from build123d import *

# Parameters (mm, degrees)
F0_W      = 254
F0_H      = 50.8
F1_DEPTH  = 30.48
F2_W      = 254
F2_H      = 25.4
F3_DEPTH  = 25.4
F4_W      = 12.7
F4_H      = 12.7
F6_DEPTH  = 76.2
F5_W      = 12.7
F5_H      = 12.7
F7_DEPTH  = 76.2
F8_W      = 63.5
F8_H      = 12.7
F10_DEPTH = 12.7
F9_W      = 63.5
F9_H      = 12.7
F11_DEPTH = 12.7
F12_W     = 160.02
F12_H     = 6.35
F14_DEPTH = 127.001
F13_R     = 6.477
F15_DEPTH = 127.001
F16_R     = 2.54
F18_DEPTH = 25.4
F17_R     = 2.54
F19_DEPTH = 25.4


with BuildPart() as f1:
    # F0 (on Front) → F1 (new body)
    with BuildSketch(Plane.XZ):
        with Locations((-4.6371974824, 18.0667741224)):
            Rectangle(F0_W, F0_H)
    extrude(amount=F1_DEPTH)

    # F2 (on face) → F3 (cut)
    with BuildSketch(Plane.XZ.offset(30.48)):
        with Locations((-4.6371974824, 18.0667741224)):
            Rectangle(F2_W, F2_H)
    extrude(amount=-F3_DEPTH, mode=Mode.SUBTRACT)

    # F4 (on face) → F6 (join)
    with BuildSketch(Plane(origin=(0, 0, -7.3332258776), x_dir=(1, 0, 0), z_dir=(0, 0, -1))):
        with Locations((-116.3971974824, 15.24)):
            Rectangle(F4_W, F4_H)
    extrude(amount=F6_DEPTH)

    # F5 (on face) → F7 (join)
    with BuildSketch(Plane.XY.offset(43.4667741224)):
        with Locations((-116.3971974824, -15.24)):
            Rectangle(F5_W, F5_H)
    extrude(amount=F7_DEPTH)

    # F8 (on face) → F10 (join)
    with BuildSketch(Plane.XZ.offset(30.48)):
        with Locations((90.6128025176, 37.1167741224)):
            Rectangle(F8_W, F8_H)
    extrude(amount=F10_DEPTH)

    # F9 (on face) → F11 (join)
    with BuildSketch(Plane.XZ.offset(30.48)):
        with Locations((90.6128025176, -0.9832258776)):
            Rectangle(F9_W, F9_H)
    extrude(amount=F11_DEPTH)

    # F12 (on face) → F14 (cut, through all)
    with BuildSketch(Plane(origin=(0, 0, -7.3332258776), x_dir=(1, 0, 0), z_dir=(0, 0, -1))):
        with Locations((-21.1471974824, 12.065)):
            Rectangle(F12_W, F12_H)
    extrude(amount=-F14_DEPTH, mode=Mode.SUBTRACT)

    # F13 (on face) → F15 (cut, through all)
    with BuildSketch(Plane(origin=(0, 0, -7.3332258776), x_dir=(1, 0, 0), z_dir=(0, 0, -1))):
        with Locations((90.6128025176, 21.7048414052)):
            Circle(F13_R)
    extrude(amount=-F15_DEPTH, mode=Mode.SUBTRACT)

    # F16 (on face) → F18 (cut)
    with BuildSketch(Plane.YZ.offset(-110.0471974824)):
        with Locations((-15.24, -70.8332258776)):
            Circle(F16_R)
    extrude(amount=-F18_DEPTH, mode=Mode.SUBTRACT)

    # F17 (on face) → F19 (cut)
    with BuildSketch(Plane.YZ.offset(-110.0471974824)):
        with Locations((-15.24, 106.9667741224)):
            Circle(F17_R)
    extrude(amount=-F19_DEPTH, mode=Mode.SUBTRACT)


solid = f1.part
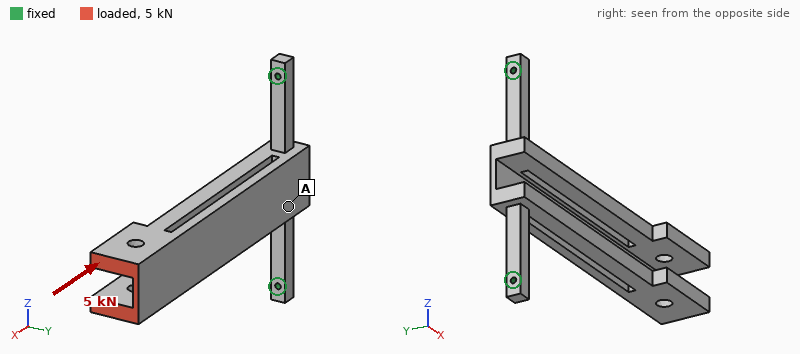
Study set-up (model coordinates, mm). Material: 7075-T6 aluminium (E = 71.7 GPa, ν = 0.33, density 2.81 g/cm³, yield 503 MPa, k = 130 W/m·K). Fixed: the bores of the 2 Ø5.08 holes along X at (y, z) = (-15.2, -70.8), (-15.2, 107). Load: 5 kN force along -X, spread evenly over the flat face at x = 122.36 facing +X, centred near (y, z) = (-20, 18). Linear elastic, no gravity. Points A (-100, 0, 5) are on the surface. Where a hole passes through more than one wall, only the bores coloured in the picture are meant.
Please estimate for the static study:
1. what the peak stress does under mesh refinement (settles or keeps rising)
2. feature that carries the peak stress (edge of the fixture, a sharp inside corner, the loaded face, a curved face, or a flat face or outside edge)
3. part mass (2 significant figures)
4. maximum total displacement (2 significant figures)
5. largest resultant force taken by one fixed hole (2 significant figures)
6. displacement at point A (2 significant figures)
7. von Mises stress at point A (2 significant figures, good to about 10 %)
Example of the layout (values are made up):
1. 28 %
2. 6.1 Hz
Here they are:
1. keeps rising
2. edge of the fixture
3. 690 g
4. 1.9 mm
5. 2.5 kN
6. 0.39 mm
7. 26 MPa
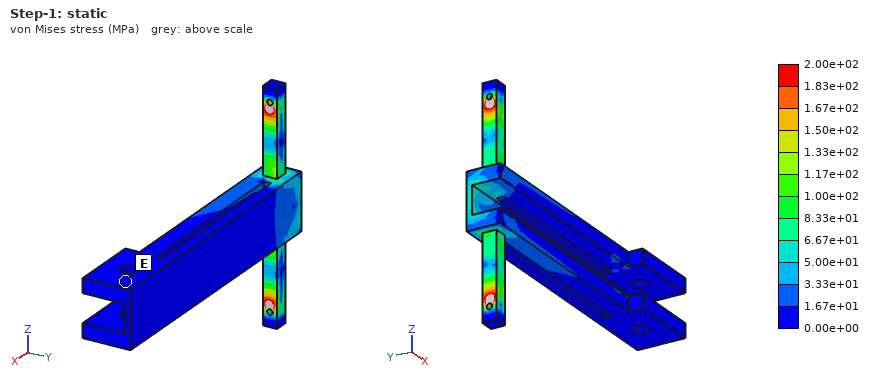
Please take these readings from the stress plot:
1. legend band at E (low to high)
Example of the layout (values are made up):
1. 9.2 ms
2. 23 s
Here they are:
1. 0.00e+00 to 1.67e+01 MPa
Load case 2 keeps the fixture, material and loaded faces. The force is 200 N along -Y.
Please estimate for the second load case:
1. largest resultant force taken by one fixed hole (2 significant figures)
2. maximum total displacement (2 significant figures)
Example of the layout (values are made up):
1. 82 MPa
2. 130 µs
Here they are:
1. 260 N
2. 3.9 mm
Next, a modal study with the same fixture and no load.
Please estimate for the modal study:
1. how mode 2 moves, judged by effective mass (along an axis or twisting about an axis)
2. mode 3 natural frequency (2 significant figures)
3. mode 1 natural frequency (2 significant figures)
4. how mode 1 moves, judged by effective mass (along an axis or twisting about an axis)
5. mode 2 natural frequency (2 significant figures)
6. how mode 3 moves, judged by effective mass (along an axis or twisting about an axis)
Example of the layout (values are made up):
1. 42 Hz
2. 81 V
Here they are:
1. along Z
2. 630 Hz
3. 76 Hz
4. along Y
5. 240 Hz
6. twisting about X
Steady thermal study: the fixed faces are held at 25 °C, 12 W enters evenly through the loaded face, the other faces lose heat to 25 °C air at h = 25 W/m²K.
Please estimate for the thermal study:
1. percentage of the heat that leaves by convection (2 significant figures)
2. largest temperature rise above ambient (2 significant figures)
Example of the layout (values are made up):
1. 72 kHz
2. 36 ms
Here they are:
1. 88 %
2. 14 K
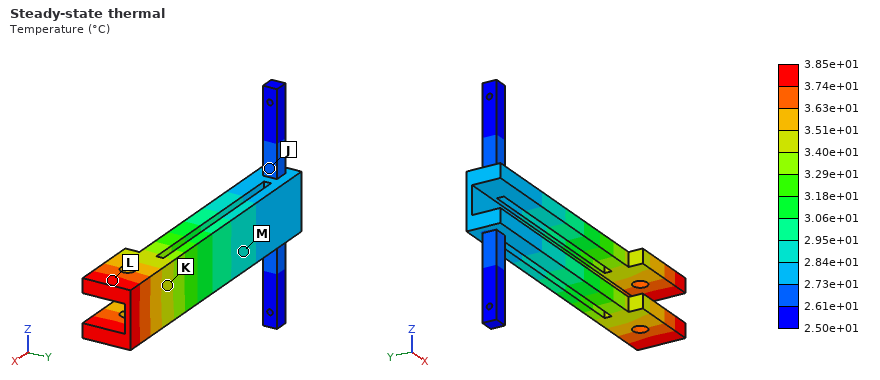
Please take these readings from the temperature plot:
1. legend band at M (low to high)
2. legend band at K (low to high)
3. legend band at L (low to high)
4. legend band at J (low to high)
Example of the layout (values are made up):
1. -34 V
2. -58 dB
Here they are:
1. 2.84e+01 to 2.95e+01 °C
2. 3.40e+01 to 3.51e+01 °C
3. 3.74e+01 to 3.85e+01 °C
4. 2.61e+01 to 2.73e+01 °C
